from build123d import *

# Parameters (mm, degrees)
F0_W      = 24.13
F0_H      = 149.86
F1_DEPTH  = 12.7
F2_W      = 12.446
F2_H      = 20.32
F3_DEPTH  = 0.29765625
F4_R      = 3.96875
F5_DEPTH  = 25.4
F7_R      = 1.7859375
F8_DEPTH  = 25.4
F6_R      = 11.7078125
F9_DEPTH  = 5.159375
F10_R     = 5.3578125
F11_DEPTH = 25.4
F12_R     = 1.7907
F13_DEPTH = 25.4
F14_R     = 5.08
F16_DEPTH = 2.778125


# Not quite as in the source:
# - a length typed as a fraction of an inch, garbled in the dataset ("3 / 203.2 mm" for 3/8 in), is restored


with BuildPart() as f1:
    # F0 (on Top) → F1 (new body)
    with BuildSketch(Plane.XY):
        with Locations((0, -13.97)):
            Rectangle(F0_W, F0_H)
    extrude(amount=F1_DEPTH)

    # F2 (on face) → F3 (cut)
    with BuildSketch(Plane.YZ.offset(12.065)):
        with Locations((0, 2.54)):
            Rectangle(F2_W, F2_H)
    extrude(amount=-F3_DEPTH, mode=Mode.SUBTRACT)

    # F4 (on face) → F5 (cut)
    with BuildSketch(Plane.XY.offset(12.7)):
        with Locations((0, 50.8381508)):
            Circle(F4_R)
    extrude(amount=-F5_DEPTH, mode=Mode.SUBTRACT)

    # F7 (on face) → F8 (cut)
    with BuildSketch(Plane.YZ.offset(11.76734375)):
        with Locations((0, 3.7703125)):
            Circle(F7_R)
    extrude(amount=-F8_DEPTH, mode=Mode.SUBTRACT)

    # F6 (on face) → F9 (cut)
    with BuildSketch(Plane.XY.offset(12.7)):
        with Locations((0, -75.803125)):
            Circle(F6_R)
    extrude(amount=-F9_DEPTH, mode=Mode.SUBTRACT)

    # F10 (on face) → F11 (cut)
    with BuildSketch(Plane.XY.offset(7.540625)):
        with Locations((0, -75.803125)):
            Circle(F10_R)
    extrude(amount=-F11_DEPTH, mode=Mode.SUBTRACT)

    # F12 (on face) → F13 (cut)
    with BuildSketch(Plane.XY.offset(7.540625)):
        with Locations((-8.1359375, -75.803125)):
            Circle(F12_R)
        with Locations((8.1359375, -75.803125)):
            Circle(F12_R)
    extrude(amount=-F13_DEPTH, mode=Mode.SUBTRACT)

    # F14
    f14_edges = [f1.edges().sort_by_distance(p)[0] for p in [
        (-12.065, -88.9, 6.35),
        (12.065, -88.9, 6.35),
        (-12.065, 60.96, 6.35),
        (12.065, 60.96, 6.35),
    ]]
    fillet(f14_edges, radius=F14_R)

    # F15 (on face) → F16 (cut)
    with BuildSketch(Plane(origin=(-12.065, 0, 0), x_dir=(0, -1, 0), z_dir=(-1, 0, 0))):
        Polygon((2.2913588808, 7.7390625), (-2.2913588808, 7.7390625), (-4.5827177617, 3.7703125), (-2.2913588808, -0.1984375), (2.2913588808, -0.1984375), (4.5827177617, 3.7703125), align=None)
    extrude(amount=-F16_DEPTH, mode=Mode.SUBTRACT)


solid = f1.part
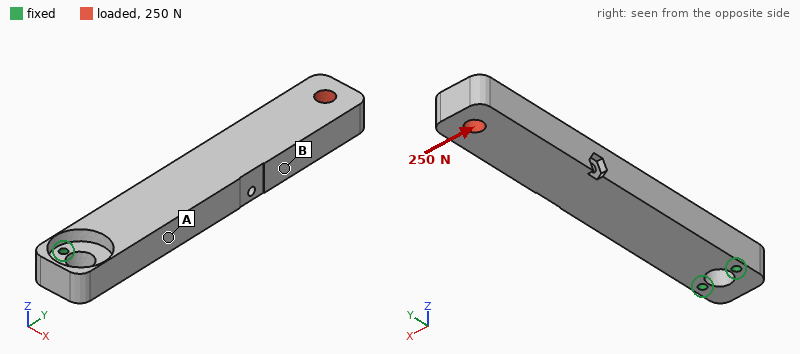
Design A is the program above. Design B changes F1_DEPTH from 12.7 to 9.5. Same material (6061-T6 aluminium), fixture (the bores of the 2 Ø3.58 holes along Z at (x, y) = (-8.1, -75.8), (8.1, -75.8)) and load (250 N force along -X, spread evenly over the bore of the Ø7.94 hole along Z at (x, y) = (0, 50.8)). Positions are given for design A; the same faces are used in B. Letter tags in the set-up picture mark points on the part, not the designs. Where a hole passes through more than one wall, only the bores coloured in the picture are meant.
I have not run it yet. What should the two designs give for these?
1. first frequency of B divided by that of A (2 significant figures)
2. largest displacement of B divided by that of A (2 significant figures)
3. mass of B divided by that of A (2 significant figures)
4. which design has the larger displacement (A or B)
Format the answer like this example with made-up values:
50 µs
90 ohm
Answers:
0.92
1.2
0.76
B
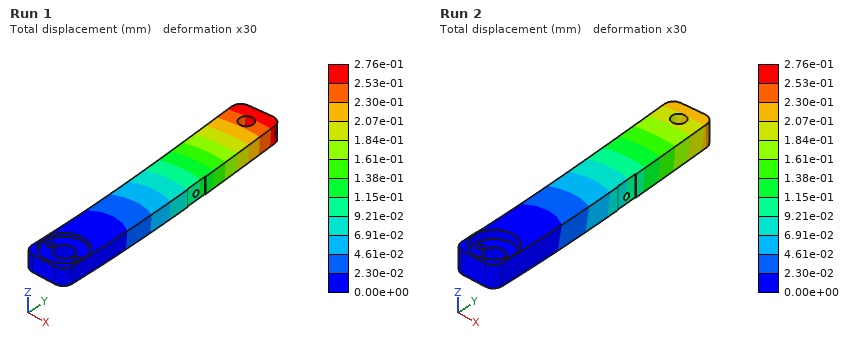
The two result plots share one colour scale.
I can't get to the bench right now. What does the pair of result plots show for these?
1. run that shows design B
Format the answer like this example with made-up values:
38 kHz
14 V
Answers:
Run 1
